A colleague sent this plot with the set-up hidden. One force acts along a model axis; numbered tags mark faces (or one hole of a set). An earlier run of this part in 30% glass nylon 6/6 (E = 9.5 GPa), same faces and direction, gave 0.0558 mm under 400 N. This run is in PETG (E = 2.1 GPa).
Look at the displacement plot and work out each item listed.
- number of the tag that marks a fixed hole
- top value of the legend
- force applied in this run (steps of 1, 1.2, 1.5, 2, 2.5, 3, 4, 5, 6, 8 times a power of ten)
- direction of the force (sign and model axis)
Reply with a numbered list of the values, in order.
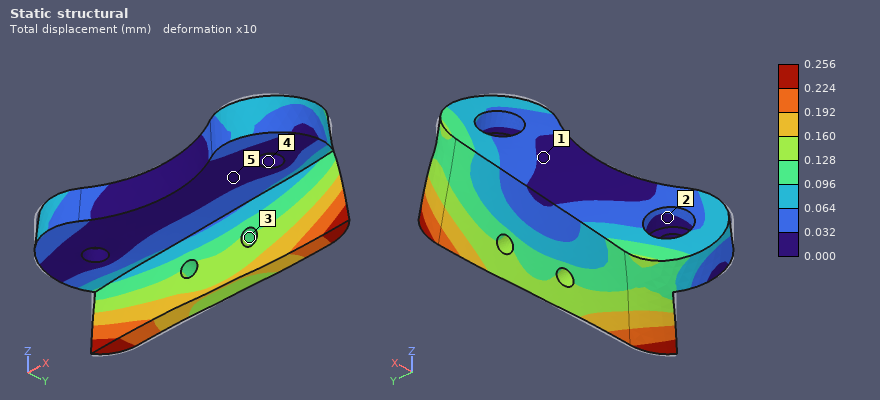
1. 4
2. 0.256 mm
3. 400 N
4. +X
